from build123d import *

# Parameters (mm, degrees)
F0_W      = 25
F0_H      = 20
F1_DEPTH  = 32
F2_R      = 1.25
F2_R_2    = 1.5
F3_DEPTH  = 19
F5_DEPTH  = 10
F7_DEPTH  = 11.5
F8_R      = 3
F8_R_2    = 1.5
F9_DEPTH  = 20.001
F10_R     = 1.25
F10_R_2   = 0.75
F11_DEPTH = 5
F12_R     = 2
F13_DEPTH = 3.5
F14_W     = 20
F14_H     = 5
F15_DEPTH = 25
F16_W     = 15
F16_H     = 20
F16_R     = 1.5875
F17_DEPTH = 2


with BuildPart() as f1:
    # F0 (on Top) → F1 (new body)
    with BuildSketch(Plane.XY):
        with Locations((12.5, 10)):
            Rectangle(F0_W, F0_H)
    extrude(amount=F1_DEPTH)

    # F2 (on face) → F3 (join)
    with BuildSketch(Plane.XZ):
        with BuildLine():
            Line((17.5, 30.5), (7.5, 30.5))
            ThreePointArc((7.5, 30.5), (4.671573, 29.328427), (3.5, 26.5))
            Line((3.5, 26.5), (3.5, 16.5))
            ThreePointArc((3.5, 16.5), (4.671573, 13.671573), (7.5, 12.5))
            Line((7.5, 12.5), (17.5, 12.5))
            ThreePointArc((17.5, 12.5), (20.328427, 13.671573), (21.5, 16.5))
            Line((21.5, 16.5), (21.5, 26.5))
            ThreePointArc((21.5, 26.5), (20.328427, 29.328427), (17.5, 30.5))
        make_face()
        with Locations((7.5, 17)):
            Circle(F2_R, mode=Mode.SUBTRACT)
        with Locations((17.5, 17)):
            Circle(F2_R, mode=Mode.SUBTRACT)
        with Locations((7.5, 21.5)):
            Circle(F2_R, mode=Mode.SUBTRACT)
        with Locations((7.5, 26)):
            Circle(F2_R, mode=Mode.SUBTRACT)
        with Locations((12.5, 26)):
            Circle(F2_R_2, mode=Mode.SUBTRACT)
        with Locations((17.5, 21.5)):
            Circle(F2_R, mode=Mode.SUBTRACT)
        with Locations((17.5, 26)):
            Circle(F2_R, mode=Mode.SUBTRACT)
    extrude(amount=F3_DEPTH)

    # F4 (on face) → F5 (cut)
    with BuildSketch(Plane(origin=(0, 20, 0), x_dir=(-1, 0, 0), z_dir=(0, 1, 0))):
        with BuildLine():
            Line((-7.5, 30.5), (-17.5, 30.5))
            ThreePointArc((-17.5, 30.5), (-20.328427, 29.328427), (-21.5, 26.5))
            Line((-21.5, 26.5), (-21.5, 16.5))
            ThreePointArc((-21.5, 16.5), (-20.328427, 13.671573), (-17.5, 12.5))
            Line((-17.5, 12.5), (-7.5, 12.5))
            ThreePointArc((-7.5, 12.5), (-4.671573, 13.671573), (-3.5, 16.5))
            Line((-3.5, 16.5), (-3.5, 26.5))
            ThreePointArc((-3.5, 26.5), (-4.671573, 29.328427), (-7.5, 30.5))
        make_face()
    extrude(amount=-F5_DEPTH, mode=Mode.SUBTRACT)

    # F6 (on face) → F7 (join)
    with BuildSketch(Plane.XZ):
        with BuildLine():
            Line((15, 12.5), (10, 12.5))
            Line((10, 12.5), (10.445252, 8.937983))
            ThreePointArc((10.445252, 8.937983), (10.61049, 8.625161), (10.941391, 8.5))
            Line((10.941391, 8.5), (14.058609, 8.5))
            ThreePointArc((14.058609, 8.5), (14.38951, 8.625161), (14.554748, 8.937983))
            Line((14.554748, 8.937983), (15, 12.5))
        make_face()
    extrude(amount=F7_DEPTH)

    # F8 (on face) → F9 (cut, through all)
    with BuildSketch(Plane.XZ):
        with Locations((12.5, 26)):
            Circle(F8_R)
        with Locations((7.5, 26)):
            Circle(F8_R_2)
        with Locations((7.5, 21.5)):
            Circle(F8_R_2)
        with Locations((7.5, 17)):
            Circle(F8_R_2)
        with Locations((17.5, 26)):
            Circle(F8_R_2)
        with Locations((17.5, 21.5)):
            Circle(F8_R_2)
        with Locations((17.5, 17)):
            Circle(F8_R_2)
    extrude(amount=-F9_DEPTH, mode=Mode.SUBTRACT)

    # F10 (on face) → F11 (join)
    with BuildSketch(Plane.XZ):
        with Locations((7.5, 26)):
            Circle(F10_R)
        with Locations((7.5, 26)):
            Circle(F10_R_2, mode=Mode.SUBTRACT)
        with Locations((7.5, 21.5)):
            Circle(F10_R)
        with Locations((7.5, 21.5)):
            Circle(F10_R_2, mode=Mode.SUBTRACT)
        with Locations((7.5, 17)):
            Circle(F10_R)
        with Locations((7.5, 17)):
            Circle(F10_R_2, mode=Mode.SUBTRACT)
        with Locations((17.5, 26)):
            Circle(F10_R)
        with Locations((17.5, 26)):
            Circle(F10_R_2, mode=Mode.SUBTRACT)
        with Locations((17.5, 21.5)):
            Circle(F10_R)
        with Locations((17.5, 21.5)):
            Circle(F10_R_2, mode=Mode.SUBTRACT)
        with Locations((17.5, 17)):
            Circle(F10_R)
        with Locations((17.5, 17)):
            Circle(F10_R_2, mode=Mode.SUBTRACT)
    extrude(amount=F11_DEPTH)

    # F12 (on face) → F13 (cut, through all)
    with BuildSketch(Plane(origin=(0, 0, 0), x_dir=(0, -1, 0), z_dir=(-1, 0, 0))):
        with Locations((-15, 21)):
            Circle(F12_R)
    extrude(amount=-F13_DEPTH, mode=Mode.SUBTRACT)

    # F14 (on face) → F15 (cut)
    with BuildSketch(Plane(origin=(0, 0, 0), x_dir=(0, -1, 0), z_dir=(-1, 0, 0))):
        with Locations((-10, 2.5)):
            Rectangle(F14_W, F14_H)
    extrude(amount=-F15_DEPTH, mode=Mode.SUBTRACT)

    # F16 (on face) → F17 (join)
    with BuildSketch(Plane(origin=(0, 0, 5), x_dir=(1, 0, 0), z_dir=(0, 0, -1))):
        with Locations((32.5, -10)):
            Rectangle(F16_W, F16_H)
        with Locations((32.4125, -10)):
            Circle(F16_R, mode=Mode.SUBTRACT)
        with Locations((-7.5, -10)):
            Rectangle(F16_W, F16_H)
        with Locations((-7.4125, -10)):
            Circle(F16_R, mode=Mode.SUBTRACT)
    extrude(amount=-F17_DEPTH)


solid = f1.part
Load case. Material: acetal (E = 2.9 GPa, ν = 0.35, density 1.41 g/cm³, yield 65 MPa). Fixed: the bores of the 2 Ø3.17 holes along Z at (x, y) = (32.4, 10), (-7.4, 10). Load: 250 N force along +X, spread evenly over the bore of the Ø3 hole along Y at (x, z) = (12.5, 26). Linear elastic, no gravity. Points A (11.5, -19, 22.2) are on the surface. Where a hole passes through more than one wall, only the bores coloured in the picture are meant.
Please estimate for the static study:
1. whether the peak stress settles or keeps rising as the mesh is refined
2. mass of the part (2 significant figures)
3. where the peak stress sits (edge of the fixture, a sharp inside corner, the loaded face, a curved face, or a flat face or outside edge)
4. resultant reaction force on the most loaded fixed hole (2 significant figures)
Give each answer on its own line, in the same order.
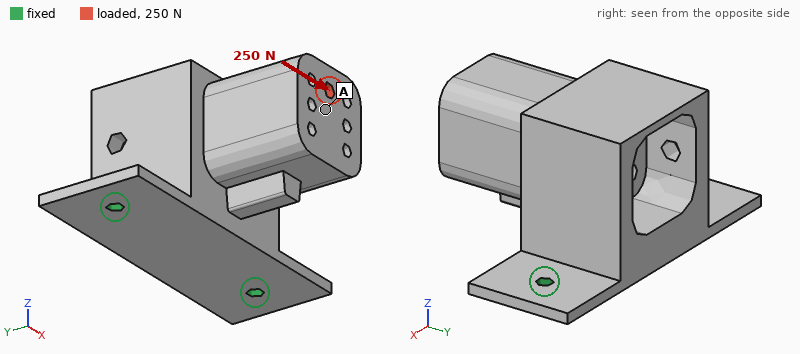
keeps rising
23 g
edge of the fixture
230 N
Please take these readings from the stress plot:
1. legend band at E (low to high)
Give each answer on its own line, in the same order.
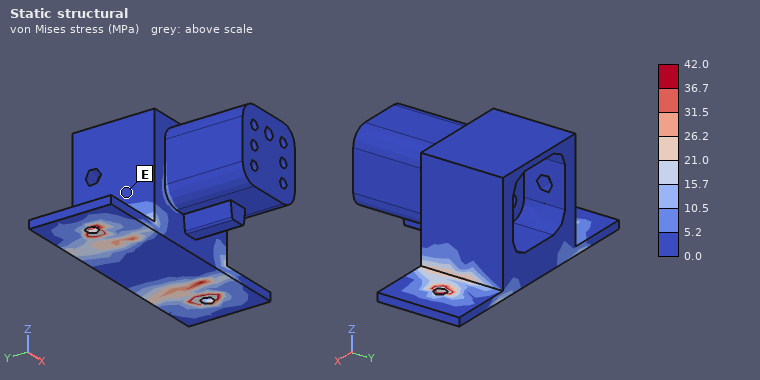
0.0 to 5.2 MPa
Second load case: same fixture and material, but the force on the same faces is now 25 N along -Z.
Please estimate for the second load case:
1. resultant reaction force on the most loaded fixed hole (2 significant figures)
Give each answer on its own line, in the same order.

14 N
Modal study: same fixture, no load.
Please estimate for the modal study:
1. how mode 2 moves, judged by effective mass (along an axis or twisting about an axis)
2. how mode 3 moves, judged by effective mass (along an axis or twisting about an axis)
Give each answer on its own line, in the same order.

along X
along Z
